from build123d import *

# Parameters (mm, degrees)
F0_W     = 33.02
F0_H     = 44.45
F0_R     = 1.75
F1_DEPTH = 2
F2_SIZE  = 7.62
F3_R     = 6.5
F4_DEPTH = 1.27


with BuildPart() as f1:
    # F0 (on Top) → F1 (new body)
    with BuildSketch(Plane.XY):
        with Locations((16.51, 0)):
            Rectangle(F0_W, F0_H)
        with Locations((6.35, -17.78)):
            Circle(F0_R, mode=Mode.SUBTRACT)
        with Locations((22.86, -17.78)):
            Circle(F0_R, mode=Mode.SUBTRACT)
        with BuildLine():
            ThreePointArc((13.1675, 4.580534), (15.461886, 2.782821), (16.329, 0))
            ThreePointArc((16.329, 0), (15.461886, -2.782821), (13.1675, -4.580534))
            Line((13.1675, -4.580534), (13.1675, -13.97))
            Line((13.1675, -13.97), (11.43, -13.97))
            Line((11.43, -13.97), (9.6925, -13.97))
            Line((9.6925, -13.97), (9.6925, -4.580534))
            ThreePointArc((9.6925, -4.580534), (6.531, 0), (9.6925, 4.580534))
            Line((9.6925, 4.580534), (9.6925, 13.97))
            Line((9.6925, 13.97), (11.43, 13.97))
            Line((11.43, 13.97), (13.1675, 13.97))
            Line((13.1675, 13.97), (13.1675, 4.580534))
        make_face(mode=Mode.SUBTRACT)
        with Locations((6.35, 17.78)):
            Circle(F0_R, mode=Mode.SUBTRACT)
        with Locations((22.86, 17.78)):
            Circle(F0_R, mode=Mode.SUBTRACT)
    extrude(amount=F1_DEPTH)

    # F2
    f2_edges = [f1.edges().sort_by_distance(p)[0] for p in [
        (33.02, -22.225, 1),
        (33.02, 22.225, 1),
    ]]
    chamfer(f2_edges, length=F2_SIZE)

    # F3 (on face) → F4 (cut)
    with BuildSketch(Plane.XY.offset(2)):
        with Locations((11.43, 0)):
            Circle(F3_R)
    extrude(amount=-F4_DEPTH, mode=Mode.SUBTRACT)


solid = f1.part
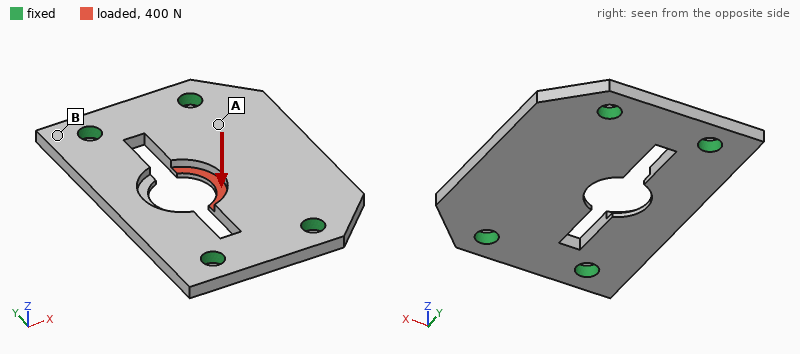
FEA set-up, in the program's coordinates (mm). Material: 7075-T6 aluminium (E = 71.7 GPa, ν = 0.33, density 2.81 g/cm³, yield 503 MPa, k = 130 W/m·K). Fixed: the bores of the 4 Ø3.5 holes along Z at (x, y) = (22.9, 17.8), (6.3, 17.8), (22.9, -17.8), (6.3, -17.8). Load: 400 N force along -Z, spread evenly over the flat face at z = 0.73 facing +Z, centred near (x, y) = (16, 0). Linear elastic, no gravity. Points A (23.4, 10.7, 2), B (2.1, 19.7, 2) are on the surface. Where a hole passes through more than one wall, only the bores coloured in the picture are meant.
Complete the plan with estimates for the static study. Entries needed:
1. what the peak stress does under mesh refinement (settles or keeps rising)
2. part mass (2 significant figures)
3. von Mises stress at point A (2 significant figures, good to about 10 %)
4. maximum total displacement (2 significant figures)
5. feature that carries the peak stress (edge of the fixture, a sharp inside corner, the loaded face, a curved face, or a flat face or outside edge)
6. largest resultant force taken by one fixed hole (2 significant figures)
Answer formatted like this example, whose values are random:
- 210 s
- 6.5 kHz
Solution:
- keeps rising
- 6.8 g
- 84 MPa
- 0.20 mm
- edge of the fixture
- 150 N
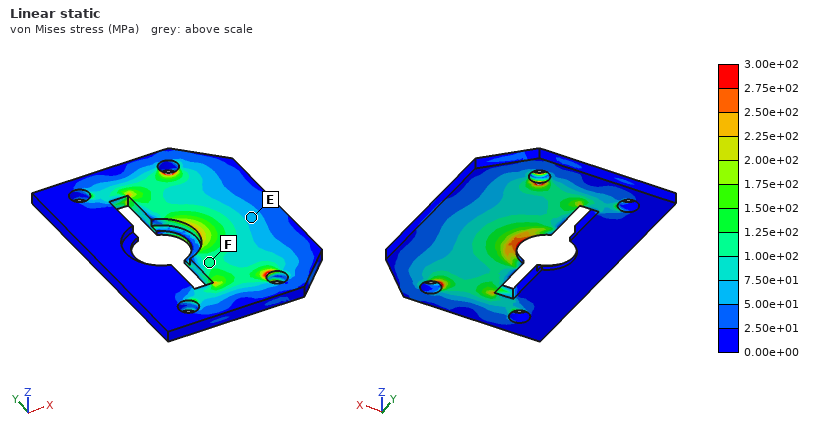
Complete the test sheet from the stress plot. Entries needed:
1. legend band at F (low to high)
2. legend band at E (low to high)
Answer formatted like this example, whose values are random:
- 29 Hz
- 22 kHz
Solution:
- 1.00e+02 to 1.25e+02 MPa
- 5.00e+01 to 7.50e+01 MPa
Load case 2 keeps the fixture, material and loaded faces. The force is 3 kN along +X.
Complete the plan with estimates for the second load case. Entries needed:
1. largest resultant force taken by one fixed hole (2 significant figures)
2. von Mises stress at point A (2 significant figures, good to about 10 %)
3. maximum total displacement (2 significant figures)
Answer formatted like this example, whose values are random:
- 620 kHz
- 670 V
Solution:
- 1.2 kN
- 72 MPa
- 69 µm
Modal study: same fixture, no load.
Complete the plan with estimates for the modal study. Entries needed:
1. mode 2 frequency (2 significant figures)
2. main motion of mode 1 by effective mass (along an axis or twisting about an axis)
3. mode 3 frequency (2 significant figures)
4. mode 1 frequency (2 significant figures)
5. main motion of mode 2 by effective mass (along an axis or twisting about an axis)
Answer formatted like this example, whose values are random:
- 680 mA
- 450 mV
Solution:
- 9400 Hz
- along Z
- 12 kHz
- 7800 Hz
- along Z
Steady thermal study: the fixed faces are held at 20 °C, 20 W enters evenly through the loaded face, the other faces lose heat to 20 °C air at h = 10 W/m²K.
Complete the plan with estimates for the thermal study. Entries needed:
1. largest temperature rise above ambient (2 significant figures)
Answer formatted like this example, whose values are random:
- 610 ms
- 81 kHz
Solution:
- 58 K
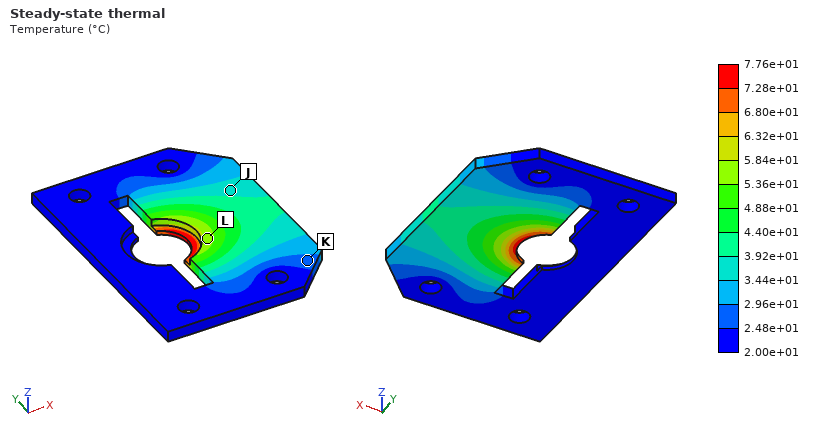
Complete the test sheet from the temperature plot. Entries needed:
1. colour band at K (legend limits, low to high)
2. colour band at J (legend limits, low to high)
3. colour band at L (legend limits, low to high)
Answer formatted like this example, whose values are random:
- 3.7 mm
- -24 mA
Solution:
- 2.48e+01 to 2.96e+01 °C
- 3.44e+01 to 3.92e+01 °C
- 5.36e+01 to 5.84e+01 °C
